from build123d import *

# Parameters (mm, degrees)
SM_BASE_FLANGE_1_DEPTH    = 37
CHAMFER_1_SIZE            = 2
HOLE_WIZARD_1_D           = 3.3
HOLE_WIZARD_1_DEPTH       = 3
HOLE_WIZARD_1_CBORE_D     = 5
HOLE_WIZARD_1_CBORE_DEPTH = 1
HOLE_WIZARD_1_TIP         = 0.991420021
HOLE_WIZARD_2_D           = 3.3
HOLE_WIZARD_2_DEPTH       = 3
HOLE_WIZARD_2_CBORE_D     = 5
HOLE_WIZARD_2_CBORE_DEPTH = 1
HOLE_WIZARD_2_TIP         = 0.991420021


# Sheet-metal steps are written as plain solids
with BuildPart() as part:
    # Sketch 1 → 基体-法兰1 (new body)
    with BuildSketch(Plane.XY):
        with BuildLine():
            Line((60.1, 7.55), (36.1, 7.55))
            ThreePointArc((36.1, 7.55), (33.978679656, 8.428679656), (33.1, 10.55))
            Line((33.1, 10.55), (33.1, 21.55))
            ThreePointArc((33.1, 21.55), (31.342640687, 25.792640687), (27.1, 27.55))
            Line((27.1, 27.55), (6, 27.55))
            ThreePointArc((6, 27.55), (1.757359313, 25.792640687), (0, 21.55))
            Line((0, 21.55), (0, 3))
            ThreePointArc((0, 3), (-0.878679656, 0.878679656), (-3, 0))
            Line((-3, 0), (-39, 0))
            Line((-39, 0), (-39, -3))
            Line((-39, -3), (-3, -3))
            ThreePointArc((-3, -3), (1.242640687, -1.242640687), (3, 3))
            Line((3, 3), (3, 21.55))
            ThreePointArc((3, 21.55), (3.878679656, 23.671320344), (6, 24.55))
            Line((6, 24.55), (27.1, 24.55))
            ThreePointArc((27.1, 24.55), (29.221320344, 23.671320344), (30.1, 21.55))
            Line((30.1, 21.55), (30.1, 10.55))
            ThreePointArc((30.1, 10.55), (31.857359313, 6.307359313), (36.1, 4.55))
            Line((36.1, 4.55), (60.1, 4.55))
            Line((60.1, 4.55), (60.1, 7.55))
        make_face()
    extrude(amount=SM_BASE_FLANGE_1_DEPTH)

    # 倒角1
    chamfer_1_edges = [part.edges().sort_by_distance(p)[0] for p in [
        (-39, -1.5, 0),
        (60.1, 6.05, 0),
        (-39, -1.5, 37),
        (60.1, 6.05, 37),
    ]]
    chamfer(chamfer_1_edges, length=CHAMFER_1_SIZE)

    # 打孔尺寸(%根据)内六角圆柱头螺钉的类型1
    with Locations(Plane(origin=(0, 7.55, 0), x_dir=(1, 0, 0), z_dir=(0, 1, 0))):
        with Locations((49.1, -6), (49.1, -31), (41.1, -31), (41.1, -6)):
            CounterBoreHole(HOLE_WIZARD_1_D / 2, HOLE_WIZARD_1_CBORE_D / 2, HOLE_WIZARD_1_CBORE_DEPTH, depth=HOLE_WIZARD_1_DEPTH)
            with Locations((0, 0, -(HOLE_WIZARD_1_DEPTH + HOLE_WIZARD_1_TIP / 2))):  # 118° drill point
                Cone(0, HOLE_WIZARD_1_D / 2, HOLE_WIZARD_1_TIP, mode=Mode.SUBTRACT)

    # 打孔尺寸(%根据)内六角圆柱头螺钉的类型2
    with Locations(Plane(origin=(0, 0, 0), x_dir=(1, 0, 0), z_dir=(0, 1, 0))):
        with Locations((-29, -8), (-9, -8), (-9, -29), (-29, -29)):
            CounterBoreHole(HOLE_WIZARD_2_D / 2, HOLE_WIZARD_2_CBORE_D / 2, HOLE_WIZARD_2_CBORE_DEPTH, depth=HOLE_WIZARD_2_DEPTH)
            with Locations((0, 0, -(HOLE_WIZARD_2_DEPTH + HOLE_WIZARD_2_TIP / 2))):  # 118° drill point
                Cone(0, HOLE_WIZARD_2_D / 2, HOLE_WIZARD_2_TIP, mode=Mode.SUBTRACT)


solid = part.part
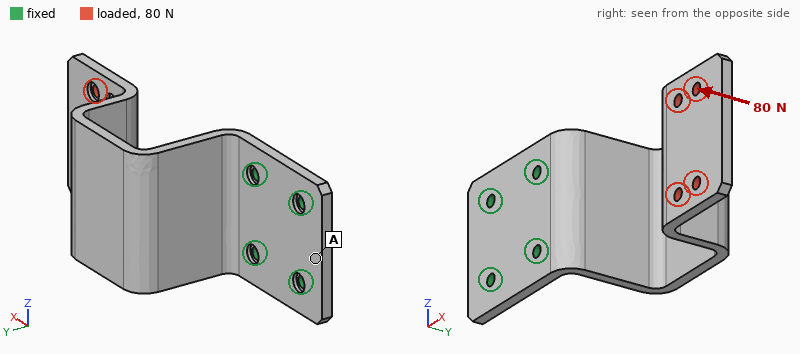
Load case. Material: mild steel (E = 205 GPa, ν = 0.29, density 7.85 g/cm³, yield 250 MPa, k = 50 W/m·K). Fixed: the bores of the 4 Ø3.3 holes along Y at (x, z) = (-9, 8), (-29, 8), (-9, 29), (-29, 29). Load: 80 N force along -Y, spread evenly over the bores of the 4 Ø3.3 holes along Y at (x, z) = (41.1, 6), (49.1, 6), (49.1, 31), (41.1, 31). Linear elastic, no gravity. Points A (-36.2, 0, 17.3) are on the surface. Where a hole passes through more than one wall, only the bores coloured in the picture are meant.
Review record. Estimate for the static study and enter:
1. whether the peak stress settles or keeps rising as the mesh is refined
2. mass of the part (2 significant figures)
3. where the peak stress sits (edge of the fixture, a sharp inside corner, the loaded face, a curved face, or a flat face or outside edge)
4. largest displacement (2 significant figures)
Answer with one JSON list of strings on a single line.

["keeps rising", "120 g", "edge of the fixture", "0.67 mm"]
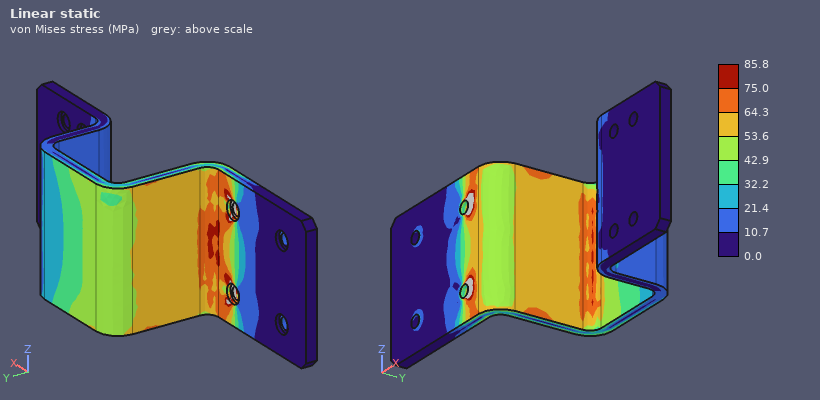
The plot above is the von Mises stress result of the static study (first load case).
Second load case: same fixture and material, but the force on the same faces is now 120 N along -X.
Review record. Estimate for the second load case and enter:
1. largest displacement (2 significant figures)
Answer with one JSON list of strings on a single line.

["0.26 mm"]
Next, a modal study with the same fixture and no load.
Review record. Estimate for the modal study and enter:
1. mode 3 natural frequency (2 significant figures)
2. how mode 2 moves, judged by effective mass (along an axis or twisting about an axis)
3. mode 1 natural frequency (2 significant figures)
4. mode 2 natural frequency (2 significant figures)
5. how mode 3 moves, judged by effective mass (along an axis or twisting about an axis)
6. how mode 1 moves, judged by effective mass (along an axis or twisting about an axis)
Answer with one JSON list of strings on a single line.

["860 Hz", "along Z", "330 Hz", "600 Hz", "along X", "along Y"]
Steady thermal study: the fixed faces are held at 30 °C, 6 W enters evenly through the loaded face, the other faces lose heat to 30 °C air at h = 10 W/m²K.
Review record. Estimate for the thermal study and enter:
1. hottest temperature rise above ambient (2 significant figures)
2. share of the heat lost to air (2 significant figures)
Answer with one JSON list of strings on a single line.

["67 K", "50 %"]
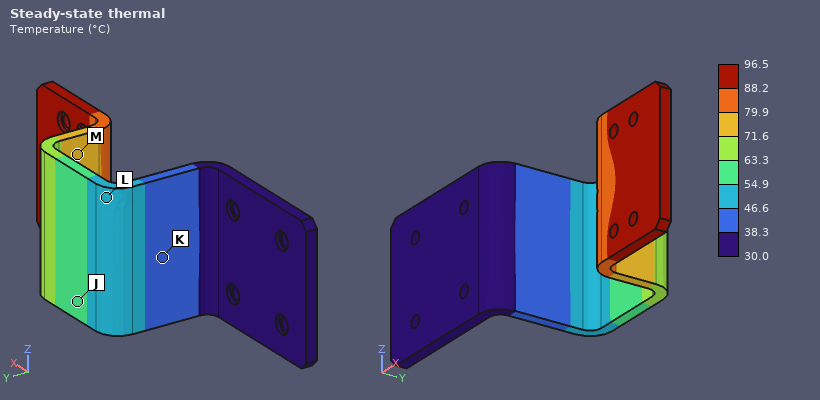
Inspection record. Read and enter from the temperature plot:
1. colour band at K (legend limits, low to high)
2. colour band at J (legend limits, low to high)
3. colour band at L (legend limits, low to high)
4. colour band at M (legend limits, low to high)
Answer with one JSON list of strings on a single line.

["38.3 to 46.6 °C", "54.9 to 63.3 °C", "46.6 to 54.9 °C", "71.6 to 79.9 °C"]
